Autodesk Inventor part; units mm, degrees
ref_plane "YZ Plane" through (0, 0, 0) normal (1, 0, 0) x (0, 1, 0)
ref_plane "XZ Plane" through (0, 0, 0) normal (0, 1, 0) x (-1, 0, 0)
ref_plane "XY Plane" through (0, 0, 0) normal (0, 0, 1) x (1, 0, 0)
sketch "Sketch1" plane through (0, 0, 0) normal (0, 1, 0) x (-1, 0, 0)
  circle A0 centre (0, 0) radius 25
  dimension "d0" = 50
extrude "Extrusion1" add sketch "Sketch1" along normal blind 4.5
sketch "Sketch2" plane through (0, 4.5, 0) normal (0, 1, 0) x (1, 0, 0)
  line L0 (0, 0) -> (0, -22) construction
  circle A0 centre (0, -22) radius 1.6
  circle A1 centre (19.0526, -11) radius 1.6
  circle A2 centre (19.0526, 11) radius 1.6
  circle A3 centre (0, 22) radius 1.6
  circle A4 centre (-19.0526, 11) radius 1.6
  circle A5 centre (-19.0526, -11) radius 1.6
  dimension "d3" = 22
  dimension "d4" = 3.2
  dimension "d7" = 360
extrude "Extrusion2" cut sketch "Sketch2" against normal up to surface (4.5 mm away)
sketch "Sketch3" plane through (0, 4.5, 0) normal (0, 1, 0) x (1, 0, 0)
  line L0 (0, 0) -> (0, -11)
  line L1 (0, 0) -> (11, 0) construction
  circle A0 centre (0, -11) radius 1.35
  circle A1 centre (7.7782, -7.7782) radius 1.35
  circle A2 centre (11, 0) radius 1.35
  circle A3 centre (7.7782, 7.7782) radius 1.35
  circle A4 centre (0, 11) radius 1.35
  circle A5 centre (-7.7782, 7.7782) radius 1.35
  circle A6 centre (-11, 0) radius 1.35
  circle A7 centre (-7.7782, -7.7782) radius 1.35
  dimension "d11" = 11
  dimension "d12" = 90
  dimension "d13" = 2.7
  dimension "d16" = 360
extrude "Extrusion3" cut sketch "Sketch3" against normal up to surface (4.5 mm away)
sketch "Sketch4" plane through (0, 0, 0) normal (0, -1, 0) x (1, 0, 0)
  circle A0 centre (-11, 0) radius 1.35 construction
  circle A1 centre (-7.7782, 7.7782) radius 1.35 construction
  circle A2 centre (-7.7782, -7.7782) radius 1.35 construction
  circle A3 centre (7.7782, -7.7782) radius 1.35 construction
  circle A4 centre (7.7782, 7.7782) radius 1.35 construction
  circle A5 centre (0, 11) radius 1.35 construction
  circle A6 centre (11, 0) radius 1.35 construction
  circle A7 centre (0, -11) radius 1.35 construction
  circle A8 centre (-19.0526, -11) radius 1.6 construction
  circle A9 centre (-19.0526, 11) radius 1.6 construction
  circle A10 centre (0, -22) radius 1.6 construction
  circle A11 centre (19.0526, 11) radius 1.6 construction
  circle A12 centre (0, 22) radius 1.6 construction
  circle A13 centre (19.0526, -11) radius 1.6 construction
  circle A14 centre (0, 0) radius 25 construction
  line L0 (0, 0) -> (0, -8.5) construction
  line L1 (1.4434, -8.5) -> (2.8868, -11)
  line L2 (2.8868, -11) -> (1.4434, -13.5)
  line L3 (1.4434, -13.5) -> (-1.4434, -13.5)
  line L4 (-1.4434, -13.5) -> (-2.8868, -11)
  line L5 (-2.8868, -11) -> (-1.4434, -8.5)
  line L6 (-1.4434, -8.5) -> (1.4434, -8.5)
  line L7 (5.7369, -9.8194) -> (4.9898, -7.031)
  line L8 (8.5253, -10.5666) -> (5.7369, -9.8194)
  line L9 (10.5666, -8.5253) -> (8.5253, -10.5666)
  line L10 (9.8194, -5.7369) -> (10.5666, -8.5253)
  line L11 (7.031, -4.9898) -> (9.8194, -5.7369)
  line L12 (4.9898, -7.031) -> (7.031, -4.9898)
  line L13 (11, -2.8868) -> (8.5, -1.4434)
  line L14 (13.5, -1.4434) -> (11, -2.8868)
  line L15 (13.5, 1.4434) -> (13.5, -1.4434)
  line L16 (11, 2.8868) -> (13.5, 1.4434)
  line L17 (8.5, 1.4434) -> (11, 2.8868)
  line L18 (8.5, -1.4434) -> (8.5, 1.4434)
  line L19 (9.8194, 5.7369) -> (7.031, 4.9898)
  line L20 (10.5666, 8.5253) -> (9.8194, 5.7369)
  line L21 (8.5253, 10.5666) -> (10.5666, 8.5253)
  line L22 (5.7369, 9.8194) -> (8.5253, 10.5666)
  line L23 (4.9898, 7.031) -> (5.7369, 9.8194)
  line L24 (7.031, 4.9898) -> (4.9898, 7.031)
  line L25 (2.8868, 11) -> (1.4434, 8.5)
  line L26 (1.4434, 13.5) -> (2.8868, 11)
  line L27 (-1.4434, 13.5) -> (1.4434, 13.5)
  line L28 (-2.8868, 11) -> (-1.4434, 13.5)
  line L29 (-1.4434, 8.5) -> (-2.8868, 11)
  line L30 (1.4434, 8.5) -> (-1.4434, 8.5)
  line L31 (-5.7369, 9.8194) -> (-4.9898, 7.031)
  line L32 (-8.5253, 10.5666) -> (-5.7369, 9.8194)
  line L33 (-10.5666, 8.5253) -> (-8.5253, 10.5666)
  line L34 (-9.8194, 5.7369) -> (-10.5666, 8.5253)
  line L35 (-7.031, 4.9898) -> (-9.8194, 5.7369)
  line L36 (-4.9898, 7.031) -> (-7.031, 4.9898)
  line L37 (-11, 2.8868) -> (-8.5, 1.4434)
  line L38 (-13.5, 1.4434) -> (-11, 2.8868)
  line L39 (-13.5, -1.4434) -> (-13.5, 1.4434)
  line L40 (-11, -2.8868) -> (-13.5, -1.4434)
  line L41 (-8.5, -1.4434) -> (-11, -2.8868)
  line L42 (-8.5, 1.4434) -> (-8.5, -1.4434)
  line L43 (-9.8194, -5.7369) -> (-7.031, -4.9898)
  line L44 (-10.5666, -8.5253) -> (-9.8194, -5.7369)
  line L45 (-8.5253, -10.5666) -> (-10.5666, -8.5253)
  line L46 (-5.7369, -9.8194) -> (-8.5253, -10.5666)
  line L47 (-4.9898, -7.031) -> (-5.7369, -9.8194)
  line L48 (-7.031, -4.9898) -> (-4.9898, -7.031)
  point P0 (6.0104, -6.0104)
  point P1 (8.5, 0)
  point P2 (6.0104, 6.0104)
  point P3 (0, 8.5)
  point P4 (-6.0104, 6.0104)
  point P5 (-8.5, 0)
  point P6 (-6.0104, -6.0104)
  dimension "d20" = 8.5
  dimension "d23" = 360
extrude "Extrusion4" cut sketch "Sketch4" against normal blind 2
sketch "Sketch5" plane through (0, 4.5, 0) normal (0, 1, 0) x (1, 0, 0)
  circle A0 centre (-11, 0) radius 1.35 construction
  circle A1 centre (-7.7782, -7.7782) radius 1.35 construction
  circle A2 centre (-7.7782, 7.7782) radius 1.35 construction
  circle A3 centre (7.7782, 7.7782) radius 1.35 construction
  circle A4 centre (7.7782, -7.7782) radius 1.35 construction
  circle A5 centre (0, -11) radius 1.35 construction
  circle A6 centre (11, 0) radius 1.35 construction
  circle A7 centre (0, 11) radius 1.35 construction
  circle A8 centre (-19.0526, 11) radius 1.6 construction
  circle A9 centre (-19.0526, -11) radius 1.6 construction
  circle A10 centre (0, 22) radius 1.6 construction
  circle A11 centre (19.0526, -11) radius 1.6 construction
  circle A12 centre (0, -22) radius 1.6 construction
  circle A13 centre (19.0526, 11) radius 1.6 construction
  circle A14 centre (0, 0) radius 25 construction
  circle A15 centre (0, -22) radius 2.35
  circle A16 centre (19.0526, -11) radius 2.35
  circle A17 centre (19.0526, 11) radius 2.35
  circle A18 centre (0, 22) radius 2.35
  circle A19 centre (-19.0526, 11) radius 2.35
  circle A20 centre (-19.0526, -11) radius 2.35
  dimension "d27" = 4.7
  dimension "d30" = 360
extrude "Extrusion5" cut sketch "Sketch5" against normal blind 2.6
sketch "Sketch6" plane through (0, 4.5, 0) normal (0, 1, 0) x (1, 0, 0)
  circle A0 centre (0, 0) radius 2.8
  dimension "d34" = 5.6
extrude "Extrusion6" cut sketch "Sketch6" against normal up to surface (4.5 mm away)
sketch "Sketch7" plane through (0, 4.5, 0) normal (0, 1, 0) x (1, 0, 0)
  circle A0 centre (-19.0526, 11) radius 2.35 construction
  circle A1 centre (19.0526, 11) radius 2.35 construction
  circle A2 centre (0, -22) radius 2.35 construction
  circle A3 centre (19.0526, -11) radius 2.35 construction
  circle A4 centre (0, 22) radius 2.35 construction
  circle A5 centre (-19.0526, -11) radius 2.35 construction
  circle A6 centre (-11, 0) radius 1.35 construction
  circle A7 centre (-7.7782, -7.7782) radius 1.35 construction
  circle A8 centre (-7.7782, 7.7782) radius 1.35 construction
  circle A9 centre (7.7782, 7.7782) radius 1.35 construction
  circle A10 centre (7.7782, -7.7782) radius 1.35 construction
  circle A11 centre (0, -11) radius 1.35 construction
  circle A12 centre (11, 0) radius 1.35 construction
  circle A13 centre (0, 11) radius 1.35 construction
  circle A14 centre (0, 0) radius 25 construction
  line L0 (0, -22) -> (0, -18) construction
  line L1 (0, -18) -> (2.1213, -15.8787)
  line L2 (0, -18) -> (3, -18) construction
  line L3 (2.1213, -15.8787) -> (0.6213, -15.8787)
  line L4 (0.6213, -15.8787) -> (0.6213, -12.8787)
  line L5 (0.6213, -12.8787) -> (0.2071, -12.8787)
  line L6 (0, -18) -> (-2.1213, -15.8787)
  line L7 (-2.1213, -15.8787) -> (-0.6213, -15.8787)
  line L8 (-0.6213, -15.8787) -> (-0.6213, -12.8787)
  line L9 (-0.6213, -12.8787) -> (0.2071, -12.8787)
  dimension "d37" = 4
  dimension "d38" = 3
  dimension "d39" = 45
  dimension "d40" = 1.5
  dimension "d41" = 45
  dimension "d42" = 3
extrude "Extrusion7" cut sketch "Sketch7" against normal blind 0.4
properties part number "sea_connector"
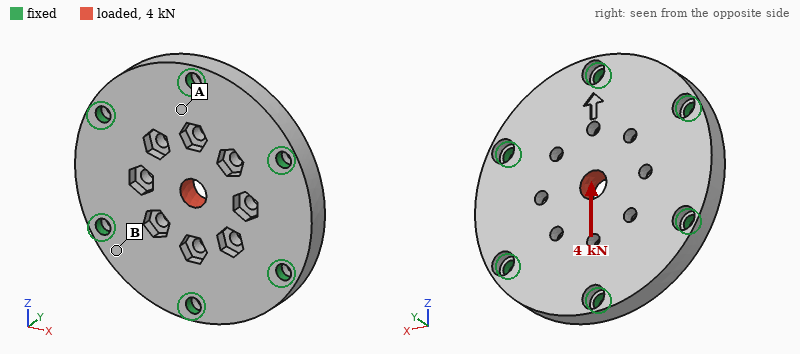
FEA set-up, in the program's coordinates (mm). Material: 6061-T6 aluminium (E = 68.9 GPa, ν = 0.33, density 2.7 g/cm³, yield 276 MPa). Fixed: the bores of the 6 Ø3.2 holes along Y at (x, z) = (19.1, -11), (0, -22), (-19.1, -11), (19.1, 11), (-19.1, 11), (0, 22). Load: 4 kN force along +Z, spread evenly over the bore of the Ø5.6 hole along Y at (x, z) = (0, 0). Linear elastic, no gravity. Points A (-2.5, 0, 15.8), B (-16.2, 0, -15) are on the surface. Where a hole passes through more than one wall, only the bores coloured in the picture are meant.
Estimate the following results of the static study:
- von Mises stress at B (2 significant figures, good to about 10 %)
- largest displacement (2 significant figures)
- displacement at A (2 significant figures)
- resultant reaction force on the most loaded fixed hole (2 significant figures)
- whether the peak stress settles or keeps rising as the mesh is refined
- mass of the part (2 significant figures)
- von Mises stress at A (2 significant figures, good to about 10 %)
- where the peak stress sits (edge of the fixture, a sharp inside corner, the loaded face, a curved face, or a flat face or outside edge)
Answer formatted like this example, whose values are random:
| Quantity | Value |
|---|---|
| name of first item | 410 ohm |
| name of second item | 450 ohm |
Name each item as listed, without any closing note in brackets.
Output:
| Quantity | Value |
|---|---|
| von Mises stress at B | 13 MPa |
| largest displacement | 13 µm |
| displacement at A | 3.9 µm |
| resultant reaction force on the most loaded fixed hole | 930 N |
| whether the peak stress settles or keeps rising as the mesh is refined | keeps rising |
| mass of the part | 21 g |
| von Mises stress at A | 33 MPa |
| where the peak stress sits | edge of the fixture |
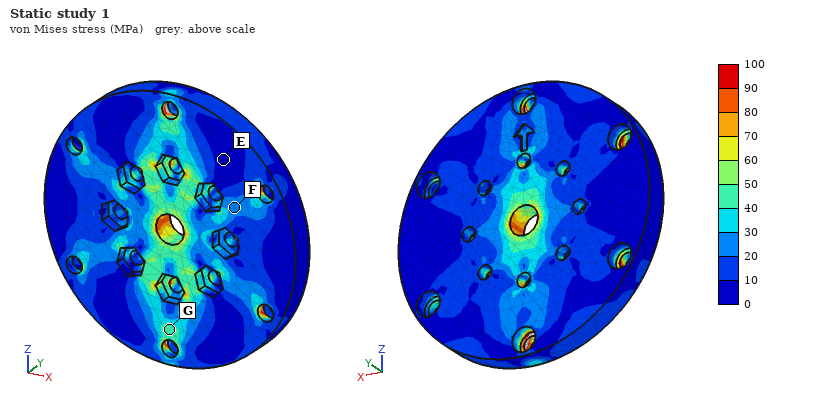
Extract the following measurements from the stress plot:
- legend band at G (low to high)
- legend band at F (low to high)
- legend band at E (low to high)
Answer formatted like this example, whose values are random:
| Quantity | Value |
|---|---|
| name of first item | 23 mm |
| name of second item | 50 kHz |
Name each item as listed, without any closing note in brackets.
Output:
| Quantity | Value |
|---|---|
| legend band at G | 40 to 50 MPa |
| legend band at F | 20 to 30 MPa |
| legend band at E | 0 to 10 MPa |
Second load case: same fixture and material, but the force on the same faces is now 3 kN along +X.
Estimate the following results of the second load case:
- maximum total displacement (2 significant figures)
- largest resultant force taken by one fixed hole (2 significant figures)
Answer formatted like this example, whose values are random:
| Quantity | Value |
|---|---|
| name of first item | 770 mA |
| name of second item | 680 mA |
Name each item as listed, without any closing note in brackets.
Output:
| Quantity | Value |
|---|---|
| maximum total displacement | 9.4 µm |
| largest resultant force taken by one fixed hole | 630 N |
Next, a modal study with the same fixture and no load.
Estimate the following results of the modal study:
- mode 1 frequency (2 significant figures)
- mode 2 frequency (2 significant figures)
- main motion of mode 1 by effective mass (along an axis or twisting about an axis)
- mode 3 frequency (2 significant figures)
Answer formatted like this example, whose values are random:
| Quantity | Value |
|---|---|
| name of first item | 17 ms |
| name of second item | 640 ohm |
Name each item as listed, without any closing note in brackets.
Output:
| Quantity | Value |
|---|---|
| mode 1 frequency | 15 kHz |
| mode 2 frequency | 27 kHz |
| main motion of mode 1 by effective mass | along Y |
| mode 3 frequency | 28 kHz |
